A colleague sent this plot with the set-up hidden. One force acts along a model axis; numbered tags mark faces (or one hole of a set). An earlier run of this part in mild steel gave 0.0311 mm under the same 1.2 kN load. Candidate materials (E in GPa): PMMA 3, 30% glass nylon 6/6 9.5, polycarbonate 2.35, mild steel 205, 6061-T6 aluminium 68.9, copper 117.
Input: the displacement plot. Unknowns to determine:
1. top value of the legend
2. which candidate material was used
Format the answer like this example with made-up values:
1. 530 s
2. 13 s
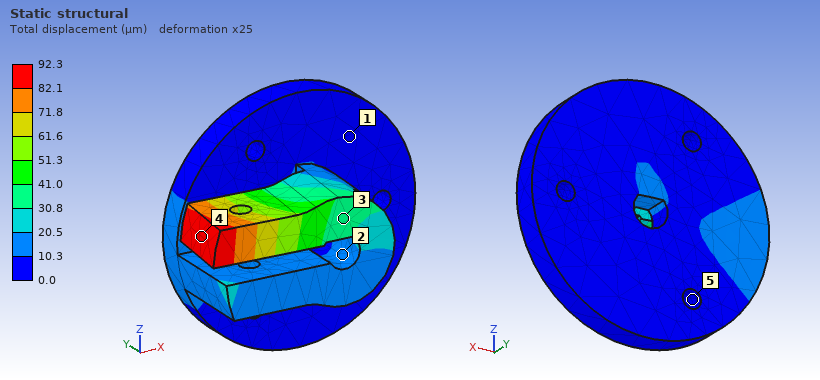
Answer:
1. 92.3 µm
2. 6061-T6 aluminium
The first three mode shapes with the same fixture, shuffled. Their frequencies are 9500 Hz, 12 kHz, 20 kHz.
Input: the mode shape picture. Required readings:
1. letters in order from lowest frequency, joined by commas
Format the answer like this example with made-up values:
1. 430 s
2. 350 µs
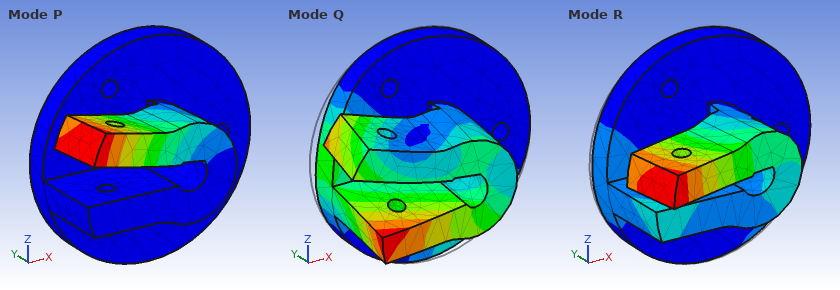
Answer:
1. P, R, Q
